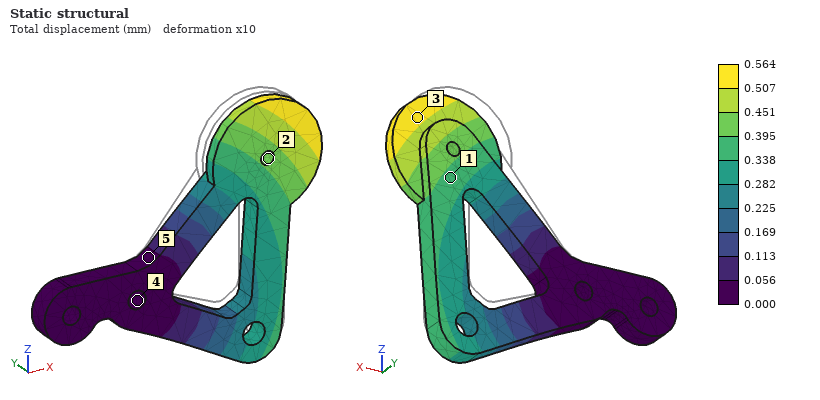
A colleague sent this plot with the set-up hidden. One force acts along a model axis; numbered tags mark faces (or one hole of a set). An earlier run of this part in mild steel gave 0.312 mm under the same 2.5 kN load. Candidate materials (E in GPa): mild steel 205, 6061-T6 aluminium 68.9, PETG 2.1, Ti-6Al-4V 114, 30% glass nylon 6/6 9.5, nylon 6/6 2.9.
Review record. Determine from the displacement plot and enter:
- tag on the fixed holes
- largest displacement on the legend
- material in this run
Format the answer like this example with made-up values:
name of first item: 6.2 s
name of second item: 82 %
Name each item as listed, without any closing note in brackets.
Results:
tag on the fixed holes: 4
largest displacement on the legend: 0.564 mm
material in this run: Ti-6Al-4V
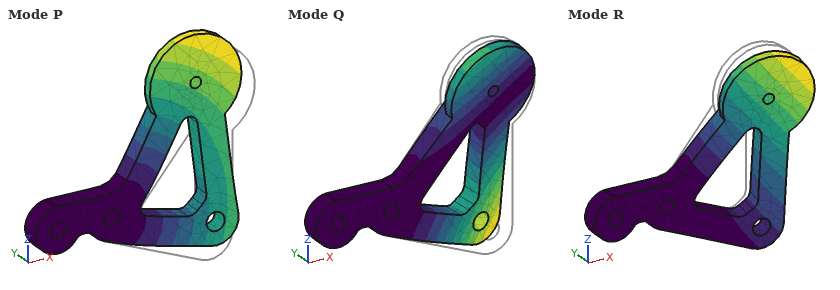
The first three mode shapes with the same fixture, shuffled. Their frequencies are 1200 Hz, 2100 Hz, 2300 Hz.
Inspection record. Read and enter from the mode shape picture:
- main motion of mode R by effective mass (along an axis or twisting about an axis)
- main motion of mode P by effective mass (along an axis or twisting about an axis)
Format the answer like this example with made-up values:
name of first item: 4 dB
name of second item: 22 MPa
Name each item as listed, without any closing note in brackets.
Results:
main motion of mode R by effective mass: along Y
main motion of mode P by effective mass: along Z
